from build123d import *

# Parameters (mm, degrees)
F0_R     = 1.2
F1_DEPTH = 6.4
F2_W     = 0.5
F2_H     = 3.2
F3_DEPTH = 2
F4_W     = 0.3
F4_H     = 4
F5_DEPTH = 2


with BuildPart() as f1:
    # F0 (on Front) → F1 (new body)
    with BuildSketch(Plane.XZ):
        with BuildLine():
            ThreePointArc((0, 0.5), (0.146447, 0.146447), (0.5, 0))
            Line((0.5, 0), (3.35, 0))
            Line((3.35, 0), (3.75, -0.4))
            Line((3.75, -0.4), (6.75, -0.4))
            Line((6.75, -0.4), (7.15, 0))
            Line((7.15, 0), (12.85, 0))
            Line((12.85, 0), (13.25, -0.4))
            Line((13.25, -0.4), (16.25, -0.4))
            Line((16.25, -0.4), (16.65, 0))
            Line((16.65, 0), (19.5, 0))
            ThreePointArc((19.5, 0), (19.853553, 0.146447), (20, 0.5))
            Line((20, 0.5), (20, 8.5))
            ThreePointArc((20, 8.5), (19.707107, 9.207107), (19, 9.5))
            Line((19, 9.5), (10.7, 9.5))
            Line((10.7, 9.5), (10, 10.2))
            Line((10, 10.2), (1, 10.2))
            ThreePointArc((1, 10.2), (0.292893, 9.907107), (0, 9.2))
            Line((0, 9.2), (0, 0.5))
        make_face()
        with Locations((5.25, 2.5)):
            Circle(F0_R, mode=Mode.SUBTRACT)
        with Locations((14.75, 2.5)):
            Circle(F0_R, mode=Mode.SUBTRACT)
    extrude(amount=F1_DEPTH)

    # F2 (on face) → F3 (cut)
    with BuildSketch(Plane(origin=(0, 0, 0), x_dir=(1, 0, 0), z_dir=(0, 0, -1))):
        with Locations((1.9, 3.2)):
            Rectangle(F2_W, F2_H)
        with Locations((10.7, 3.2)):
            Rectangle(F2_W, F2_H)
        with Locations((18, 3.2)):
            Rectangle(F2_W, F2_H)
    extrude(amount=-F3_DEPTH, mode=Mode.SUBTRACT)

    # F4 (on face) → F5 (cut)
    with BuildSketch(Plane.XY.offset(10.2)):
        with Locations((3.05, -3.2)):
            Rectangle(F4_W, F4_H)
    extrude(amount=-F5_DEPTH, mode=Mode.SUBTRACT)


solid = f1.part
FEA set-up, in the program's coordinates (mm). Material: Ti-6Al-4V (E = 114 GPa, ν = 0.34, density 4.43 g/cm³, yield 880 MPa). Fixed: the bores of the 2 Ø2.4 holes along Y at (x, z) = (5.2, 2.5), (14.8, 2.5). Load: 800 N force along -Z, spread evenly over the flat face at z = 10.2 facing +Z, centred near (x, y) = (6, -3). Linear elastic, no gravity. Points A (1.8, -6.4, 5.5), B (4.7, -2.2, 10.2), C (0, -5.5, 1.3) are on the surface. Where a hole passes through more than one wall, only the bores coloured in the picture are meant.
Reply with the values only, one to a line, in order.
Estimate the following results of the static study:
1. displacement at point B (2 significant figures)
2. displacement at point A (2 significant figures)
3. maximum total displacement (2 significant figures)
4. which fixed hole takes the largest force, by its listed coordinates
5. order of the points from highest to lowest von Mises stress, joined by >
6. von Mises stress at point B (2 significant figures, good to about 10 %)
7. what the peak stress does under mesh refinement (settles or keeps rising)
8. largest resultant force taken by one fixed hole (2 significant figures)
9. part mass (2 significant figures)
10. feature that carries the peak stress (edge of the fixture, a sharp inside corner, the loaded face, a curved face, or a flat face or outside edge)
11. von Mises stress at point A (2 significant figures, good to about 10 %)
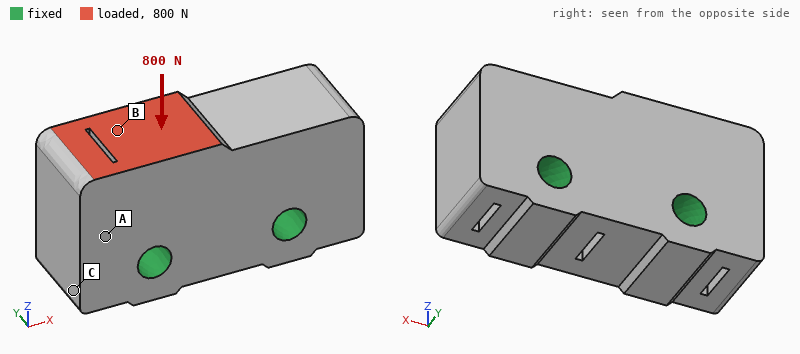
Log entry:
1.2 µm
0.90 µm
1.4 µm
(5.2, 2.5)
B > A > C
14 MPa
keeps rising
730 N
5.3 g
edge of the fixture
8.3 MPa
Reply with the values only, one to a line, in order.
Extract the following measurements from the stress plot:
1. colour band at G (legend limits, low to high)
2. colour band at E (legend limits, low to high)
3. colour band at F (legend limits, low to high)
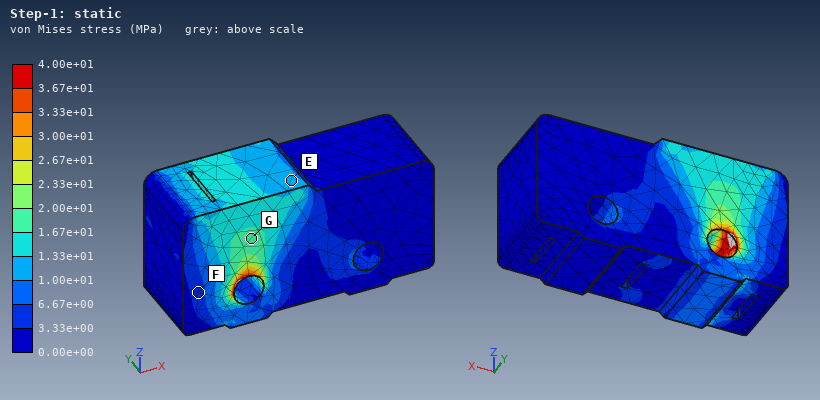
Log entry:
1.67e+01 to 2.00e+01 MPa
1.00e+01 to 1.33e+01 MPa
3.33e+00 to 6.67e+00 MPa
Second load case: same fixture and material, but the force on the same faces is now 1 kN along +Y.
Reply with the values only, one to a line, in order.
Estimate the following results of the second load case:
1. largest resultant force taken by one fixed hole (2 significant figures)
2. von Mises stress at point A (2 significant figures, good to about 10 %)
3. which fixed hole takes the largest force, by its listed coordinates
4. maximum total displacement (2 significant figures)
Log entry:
810 N
40 MPa
(5.2, 2.5)
10 µm
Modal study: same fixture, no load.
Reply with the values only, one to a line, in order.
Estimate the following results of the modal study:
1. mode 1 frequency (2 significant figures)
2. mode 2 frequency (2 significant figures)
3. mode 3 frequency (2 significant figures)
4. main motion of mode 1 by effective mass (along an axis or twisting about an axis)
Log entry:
60 kHz
69 kHz
72 kHz
along Y
